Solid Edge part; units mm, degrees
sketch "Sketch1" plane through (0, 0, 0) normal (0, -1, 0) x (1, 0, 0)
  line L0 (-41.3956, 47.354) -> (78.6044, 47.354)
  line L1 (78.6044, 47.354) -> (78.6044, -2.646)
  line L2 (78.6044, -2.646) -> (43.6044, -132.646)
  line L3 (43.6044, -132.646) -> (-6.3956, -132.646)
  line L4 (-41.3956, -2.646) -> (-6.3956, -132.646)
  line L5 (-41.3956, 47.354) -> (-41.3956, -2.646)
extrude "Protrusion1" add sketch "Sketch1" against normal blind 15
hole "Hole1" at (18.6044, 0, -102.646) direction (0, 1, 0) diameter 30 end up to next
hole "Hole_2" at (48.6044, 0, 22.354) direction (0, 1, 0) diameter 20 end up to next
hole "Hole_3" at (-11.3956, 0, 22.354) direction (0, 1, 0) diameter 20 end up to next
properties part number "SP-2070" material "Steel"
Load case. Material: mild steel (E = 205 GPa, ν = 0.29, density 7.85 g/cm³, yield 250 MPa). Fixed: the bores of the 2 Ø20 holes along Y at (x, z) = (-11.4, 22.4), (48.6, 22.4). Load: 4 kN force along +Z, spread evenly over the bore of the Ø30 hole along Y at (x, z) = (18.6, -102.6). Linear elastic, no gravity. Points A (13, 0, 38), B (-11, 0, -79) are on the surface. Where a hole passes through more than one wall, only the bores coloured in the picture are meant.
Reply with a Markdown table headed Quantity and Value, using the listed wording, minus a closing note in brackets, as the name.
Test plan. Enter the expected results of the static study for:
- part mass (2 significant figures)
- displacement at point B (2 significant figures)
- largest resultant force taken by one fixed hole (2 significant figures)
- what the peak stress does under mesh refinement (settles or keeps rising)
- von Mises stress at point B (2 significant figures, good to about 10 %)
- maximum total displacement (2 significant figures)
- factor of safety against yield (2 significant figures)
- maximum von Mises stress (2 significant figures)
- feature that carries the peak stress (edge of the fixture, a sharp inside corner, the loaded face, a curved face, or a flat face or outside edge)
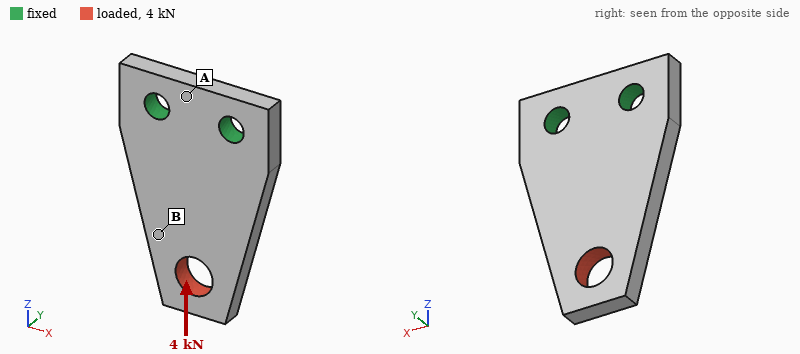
| Quantity | Value |
|---|---|
| part mass | 1.9 kg |
| displacement at point B | 1.4 µm |
| largest resultant force taken by one fixed hole | 2.0 kN |
| what the peak stress does under mesh refinement | settles |
| von Mises stress at point B | 3.7 MPa |
| maximum total displacement | 2.9 µm |
| factor of safety against yield | 25 |
| maximum von Mises stress | 9.8 MPa |
| feature that carries the peak stress | the loaded face |
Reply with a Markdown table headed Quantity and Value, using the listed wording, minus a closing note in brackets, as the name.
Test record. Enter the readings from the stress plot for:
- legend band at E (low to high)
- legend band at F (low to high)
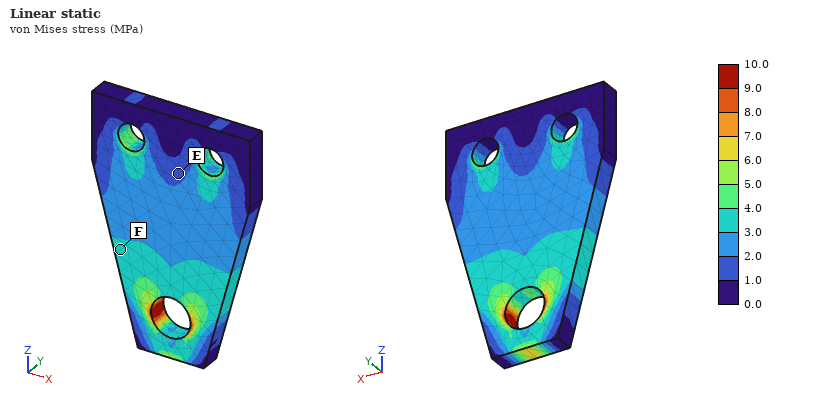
| Quantity | Value |
|---|---|
| legend band at E | 1.0 to 2.0 MPa |
| legend band at F | 3.0 to 4.0 MPa |
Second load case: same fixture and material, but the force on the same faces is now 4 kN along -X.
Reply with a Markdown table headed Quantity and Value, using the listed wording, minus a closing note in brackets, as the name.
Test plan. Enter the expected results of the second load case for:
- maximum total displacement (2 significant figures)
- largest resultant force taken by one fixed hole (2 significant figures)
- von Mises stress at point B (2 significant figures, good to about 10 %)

| Quantity | Value |
|---|---|
| maximum total displacement | 19 µm |
| largest resultant force taken by one fixed hole | 6.8 kN |
| von Mises stress at point B | 5.9 MPa |
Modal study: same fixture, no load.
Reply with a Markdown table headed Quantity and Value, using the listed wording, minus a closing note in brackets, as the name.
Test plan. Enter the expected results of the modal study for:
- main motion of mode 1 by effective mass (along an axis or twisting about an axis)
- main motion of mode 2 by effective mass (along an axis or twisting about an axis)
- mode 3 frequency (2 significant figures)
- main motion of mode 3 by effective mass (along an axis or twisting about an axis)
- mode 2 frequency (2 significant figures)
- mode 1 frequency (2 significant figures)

| Quantity | Value |
|---|---|
| main motion of mode 1 by effective mass | along Y |
| main motion of mode 2 by effective mass | twisting about Z |
| mode 3 frequency | 3400 Hz |
| main motion of mode 3 by effective mass | along Y |
| mode 2 frequency | 2700 Hz |
| mode 1 frequency | 770 Hz |
